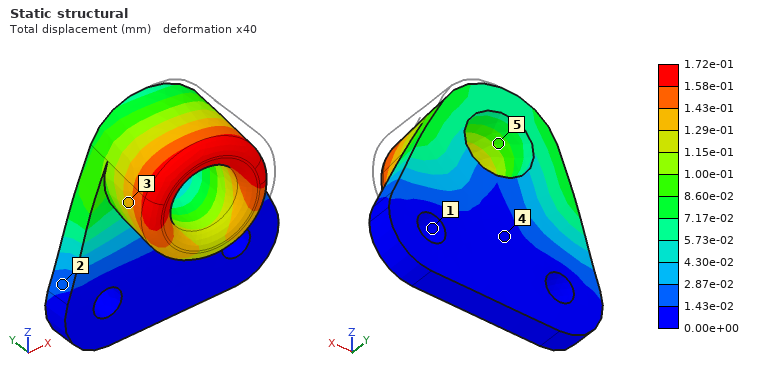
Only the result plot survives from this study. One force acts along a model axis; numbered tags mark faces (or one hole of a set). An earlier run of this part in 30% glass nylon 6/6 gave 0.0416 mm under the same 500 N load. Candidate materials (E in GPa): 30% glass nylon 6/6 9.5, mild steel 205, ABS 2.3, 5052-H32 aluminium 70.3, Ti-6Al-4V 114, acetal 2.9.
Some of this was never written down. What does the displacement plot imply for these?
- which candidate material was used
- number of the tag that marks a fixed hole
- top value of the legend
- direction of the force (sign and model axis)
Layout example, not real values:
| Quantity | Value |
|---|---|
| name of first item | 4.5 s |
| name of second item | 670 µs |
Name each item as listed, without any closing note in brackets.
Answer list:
| Quantity | Value |
|---|---|
| which candidate material was used | ABS |
| number of the tag that marks a fixed hole | 1 |
| top value of the legend | 1.72e-01 mm |
| direction of the force | -X |
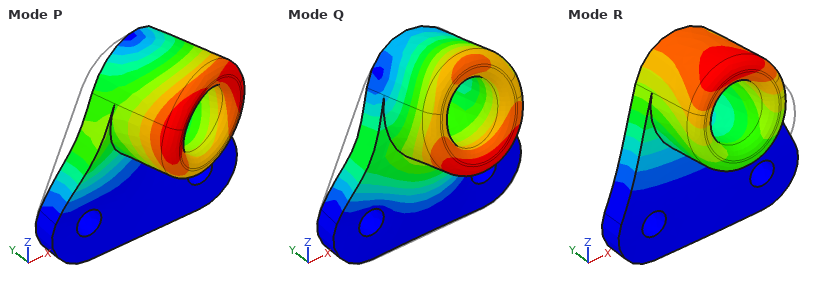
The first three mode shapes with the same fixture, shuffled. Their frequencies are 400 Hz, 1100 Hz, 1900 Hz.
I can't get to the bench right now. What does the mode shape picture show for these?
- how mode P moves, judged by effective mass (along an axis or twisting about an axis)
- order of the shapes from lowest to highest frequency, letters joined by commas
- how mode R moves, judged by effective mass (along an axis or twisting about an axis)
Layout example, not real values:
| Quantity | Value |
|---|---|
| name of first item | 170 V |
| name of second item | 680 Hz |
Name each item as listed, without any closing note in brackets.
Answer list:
| Quantity | Value |
|---|---|
| how mode P moves, judged by effective mass | along X |
| order of the shapes from lowest to highest frequency, letters joined by commas | R, P, Q |
| how mode R moves, judged by effective mass | along Y |
